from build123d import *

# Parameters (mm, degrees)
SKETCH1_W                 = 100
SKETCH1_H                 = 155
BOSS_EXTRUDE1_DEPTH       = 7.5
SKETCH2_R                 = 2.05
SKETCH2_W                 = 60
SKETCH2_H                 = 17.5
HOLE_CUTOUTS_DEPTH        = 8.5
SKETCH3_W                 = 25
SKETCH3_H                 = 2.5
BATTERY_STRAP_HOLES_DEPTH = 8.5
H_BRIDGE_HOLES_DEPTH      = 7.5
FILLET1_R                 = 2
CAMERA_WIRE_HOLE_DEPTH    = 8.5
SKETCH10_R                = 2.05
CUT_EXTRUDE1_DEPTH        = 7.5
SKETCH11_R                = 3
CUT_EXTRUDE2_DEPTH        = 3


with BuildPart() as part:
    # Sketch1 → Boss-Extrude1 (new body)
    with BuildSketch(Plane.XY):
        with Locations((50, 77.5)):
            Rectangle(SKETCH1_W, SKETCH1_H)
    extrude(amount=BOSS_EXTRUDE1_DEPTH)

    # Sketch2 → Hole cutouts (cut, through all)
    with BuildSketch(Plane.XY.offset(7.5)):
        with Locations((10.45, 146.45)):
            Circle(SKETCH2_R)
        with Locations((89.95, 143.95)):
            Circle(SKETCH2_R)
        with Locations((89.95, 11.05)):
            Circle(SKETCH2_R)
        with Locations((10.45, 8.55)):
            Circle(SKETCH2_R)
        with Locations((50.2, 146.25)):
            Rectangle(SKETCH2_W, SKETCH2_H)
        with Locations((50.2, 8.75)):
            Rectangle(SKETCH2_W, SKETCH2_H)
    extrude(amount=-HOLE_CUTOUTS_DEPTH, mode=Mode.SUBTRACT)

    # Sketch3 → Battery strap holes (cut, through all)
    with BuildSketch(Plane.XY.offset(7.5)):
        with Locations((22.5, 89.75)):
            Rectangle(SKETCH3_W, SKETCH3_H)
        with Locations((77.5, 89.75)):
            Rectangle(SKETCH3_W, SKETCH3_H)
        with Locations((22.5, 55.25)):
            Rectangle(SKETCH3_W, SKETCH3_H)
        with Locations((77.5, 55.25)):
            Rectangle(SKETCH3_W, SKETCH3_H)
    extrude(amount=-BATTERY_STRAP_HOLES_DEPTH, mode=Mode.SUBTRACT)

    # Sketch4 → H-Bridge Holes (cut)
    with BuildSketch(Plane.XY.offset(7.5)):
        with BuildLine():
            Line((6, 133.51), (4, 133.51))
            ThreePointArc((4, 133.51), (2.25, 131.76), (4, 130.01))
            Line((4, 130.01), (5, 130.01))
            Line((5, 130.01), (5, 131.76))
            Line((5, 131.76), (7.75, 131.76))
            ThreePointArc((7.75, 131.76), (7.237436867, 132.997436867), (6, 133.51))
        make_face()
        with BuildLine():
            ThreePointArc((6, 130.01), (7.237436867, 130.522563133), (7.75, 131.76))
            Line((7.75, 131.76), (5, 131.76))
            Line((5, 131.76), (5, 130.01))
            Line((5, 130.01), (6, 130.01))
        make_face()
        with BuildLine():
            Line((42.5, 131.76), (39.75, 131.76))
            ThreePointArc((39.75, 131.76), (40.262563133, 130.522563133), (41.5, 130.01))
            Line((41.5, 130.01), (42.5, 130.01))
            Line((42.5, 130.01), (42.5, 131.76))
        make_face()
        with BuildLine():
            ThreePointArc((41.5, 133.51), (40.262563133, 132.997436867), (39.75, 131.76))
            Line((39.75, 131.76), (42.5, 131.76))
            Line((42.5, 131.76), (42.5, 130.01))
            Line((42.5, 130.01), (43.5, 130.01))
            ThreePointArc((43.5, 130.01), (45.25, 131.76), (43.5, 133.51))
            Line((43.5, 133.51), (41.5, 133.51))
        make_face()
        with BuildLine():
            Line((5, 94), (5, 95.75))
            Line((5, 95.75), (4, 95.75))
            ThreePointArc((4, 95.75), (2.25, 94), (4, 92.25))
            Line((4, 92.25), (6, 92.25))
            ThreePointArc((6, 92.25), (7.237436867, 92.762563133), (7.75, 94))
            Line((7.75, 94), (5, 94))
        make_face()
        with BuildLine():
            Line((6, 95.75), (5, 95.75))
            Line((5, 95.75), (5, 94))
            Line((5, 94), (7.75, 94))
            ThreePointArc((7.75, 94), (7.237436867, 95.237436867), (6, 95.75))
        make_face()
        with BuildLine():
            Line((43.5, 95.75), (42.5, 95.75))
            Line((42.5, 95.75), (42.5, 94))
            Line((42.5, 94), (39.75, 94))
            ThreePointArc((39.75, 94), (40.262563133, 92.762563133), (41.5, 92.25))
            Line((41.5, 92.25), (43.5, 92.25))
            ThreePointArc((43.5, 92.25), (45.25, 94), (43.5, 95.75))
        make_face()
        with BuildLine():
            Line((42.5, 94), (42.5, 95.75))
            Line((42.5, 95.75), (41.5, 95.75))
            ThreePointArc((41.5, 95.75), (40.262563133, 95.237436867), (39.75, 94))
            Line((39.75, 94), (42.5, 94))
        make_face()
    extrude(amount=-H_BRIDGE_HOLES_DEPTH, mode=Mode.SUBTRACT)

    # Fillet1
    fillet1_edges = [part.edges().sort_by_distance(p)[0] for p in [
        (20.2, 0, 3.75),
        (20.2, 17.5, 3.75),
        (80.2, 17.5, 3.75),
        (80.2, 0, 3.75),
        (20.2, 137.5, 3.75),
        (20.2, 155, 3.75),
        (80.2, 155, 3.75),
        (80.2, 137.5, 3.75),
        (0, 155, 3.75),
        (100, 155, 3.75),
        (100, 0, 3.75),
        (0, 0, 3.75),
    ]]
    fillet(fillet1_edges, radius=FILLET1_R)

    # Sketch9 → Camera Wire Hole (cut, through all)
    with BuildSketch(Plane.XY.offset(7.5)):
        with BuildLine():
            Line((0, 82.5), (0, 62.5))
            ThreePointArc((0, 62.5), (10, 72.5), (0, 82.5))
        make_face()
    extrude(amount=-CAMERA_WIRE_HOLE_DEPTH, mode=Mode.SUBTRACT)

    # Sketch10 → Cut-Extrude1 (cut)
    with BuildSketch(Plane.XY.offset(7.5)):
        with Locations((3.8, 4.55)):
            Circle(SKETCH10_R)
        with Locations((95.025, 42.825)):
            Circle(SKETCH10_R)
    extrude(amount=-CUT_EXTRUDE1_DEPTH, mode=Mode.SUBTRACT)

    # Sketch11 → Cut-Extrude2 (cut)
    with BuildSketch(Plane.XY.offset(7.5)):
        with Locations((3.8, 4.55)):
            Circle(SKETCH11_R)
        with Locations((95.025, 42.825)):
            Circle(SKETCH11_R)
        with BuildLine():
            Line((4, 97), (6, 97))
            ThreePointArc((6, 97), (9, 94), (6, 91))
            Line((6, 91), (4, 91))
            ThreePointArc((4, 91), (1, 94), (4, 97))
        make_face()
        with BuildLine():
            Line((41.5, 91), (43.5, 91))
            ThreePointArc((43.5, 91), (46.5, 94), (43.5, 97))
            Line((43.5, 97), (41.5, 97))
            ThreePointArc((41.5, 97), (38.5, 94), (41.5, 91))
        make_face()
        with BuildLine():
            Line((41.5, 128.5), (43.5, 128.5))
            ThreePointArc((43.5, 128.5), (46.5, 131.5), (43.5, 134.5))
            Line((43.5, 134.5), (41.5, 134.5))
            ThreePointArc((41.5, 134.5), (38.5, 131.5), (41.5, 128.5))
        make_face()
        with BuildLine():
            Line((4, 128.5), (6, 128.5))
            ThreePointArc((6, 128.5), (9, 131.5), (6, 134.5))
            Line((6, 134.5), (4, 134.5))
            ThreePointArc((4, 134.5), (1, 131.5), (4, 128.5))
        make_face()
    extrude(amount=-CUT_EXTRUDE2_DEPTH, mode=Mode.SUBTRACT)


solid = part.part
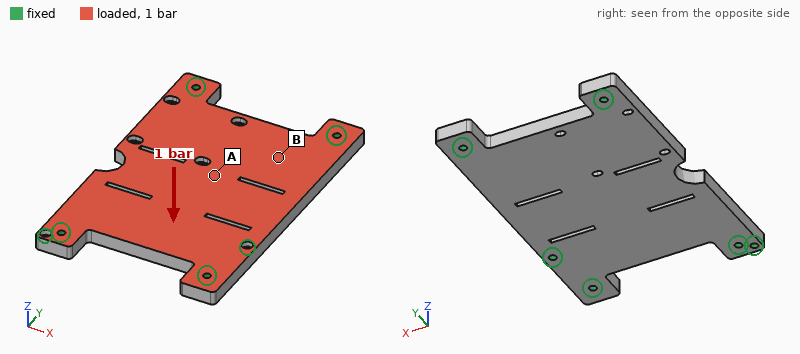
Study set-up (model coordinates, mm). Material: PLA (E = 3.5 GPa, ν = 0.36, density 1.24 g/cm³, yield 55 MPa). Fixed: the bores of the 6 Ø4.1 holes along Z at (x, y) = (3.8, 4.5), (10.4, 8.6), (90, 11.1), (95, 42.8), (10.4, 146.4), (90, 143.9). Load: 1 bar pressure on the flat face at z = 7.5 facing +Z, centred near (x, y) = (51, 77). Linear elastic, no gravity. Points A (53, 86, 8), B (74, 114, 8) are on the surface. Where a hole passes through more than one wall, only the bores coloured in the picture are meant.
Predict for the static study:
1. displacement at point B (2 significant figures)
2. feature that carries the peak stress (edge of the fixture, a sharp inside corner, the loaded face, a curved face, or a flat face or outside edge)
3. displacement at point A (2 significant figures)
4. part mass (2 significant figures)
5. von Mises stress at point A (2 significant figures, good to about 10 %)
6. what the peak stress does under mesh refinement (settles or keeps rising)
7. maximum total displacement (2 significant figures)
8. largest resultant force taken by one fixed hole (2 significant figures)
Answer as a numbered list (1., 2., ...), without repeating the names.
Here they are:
1. 0.54 mm
2. edge of the fixture
3. 1.0 mm
4. 120 g
5. 11 MPa
6. keeps rising
7. 1.4 mm
8. 440 N
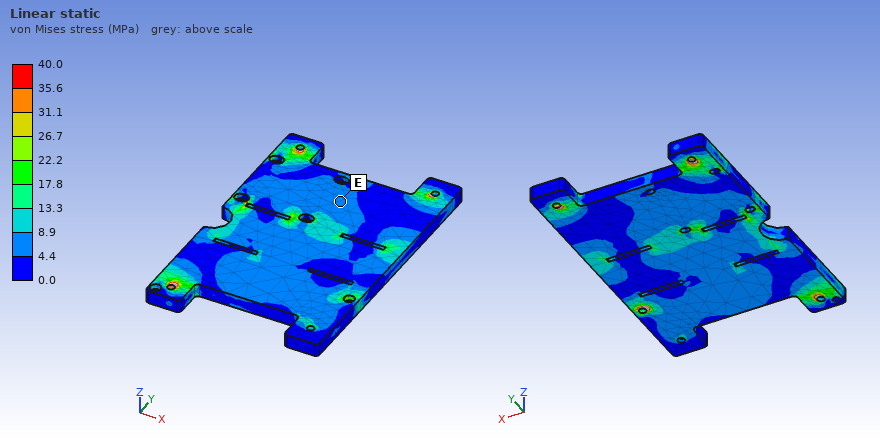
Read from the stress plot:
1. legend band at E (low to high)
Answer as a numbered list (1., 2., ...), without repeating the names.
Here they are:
1. 4.4 to 8.9 MPa
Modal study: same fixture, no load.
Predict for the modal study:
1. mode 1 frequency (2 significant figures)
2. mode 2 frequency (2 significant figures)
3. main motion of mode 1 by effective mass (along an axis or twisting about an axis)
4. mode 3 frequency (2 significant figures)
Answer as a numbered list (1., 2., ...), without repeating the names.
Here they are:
1. 560 Hz
2. 1100 Hz
3. along Z
4. 1400 Hz
